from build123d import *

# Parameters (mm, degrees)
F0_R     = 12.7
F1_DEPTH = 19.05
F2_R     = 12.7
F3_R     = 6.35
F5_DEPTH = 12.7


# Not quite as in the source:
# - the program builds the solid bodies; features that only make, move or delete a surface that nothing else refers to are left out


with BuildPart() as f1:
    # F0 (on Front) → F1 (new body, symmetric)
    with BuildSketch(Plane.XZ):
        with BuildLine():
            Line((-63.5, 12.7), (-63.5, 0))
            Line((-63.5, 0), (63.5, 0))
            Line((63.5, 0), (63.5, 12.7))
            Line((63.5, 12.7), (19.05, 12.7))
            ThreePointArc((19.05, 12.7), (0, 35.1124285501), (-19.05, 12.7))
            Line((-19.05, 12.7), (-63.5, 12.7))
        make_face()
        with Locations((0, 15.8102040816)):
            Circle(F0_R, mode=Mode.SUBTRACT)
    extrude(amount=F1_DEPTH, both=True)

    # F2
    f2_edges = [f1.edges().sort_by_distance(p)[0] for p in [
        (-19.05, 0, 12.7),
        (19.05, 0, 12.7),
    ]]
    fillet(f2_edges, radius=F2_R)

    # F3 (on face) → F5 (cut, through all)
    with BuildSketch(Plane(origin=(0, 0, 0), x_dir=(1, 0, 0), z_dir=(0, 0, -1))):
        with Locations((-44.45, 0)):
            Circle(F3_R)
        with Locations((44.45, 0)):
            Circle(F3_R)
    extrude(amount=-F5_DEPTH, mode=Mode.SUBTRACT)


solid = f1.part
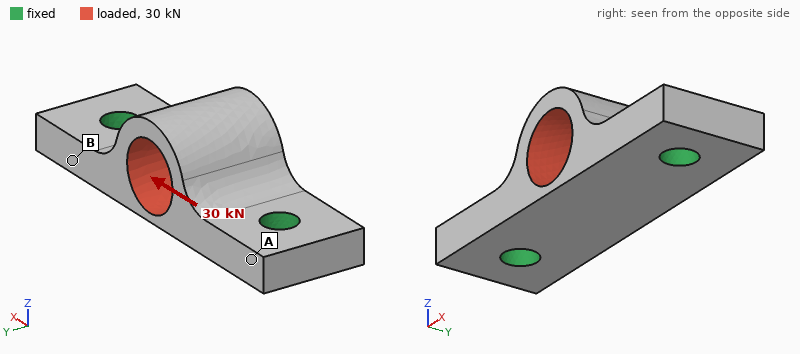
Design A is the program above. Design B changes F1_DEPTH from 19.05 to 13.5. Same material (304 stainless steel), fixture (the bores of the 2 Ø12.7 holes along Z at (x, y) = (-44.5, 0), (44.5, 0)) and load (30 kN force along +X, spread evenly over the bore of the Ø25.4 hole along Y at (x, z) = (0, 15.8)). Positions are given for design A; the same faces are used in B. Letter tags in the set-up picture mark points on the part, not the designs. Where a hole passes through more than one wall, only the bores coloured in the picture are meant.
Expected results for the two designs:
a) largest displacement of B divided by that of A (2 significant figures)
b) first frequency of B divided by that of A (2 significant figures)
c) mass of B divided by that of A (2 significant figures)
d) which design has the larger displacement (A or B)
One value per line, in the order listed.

1.4
1.0
0.69
B
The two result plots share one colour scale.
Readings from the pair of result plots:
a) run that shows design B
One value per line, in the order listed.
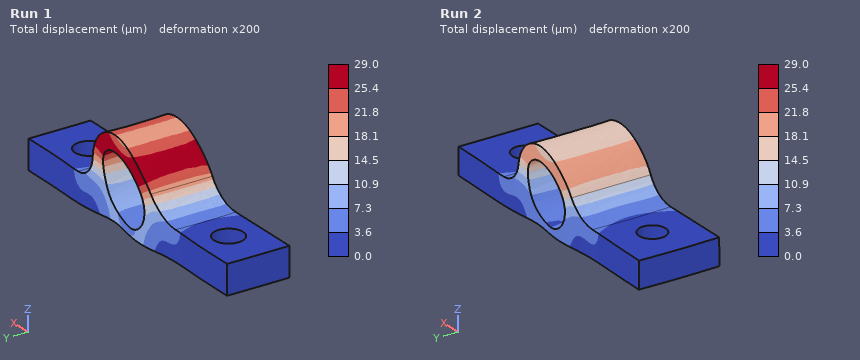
Run 1
